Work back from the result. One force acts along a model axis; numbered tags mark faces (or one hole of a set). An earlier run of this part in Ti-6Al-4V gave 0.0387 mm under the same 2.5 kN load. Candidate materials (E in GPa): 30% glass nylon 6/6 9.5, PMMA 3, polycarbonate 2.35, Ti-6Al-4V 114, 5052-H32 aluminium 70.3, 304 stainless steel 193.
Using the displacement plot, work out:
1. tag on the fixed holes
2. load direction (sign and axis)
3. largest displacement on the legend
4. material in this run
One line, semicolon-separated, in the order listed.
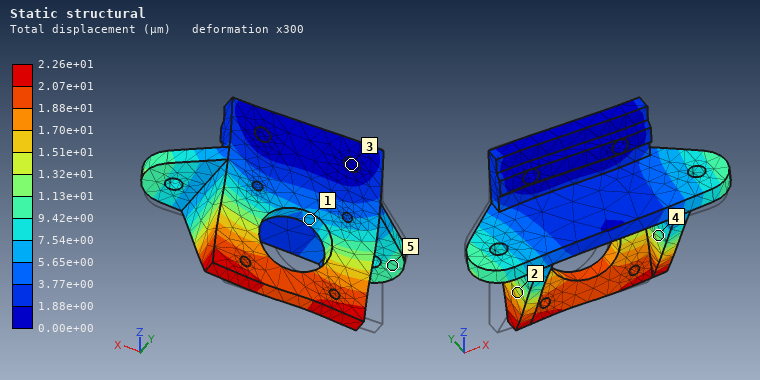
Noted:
3; +X; 2.26e+01 µm; 304 stainless steel
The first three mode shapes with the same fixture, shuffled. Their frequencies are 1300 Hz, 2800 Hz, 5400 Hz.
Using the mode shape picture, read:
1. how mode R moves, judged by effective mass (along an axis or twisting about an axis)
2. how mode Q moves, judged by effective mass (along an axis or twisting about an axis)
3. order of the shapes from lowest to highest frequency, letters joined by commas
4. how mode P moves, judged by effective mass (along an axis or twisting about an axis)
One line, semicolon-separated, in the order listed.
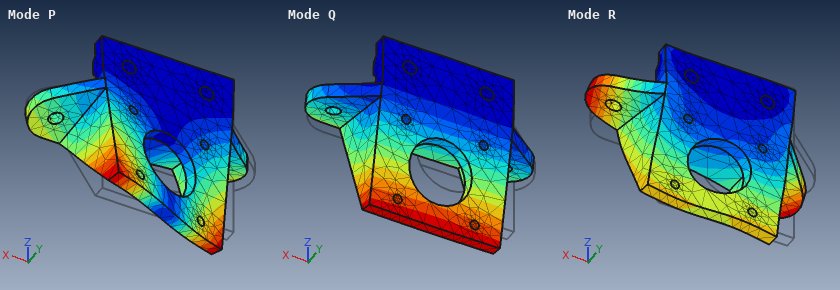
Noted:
along X; along Y; Q, P, R; twisting about Z
